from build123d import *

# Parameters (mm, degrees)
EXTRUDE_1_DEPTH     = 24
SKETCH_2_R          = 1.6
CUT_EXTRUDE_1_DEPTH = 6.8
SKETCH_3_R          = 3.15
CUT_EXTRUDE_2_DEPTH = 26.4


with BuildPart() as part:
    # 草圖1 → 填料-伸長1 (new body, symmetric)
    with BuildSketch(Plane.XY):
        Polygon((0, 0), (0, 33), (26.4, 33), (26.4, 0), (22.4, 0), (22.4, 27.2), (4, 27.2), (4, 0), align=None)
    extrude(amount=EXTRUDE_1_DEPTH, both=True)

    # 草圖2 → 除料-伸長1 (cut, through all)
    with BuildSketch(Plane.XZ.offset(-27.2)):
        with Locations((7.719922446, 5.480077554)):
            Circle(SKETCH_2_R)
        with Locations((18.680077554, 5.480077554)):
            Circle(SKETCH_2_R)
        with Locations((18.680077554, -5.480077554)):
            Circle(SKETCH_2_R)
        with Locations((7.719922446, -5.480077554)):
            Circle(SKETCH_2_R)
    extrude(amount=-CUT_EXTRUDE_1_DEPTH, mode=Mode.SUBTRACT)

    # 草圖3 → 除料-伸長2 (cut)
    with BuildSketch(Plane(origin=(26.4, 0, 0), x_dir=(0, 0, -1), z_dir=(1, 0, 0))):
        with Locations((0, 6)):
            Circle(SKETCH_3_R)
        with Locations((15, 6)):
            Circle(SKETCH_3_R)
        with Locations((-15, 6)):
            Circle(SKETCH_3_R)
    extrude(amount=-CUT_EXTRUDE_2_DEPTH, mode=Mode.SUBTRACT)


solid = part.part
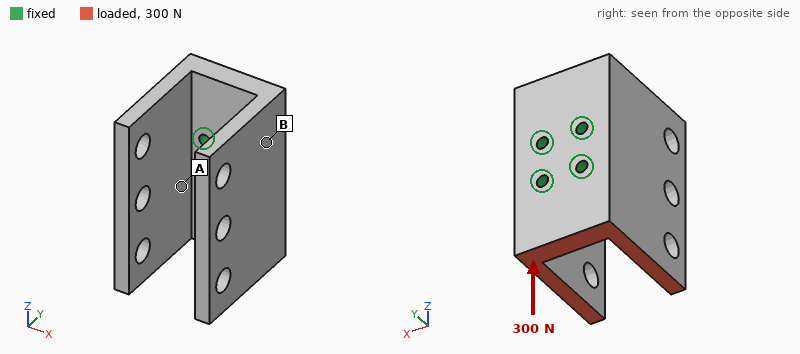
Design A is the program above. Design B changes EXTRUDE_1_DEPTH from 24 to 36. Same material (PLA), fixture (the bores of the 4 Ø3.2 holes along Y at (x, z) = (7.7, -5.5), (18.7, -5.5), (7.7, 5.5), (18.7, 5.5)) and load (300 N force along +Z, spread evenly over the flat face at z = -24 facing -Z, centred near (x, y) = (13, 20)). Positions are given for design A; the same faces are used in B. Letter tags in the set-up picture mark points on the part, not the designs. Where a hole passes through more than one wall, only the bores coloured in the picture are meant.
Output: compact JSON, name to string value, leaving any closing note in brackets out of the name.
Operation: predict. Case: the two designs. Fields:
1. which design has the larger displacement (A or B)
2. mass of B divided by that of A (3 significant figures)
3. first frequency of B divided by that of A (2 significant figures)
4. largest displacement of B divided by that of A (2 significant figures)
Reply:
{"which design has the larger displacement": "B", "mass of B divided by that of A": "1.53", "first frequency of B divided by that of A": "0.93", "largest displacement of B divided by that of A": "1.2"}
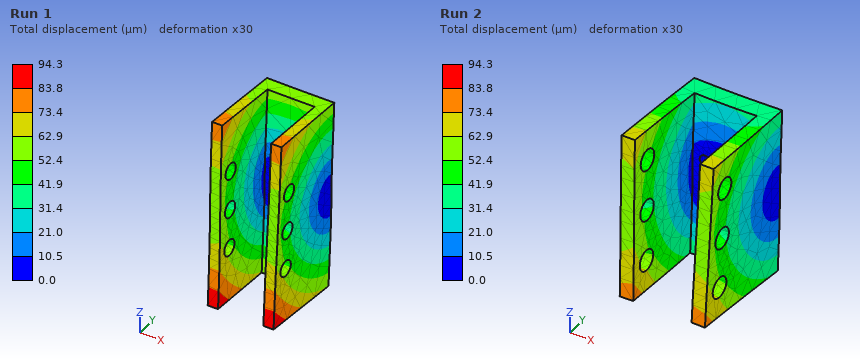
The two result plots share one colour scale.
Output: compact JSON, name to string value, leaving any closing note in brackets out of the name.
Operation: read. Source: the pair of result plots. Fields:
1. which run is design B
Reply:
{"which run is design B": "Run 1"}
